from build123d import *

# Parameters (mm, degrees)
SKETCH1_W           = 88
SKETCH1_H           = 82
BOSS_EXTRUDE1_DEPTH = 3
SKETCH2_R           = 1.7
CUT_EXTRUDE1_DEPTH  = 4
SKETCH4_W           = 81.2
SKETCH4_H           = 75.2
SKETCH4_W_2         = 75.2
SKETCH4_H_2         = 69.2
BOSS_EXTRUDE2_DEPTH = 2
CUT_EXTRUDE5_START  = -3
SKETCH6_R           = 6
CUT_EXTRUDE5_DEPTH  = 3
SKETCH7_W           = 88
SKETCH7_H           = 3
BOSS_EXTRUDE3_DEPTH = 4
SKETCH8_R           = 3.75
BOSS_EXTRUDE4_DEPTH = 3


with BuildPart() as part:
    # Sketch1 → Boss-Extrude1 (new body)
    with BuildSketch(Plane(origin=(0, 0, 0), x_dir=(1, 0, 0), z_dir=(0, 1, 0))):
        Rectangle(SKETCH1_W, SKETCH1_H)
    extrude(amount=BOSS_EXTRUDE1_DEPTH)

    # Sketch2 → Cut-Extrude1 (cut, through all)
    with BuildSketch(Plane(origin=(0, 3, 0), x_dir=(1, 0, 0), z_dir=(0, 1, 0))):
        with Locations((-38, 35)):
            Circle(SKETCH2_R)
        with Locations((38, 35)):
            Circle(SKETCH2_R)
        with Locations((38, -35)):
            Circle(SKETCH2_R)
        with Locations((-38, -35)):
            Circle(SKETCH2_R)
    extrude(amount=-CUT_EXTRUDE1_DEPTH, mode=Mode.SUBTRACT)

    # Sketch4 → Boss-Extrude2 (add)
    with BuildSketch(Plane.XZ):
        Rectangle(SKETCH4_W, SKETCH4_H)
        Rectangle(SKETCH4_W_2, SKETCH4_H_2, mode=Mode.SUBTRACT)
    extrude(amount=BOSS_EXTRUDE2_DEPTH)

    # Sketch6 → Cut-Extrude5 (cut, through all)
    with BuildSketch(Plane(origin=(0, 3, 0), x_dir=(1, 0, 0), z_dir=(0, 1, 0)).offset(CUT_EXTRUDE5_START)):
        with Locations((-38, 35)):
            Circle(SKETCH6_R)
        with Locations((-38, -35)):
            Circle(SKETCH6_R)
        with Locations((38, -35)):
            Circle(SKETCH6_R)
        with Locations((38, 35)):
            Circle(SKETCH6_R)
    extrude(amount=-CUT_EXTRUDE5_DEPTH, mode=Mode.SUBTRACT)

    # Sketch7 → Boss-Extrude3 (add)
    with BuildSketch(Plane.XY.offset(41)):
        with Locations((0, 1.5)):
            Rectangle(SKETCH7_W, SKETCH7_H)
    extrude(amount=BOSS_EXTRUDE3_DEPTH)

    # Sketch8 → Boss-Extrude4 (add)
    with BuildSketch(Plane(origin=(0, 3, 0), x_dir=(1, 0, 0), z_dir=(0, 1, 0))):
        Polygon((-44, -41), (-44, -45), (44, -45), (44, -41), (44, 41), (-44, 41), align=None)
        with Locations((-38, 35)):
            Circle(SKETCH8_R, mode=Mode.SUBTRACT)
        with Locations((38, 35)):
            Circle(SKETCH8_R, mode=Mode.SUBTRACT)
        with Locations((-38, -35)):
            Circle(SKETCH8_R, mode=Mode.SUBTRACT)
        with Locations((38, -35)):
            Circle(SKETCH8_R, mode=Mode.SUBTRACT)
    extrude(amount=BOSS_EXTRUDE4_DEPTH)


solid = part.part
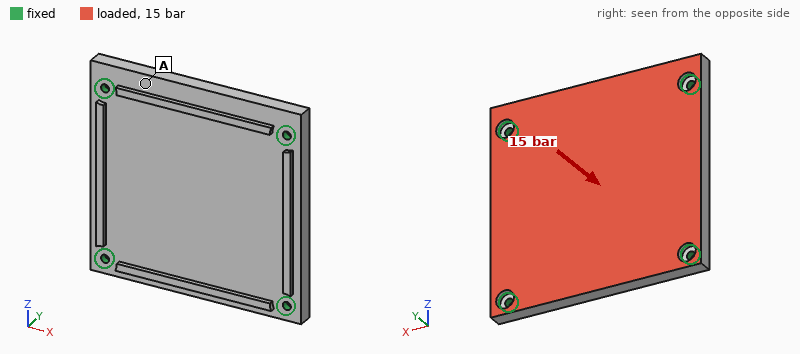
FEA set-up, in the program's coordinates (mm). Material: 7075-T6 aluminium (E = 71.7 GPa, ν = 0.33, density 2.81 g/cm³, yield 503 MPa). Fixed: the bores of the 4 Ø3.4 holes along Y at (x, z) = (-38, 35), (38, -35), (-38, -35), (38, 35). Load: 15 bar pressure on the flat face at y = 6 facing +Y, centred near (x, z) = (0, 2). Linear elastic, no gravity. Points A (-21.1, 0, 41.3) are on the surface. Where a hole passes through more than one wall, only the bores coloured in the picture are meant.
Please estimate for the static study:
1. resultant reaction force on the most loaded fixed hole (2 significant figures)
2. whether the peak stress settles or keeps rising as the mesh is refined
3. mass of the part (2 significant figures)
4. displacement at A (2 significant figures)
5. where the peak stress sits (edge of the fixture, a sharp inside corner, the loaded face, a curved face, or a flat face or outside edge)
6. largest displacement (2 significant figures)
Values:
4.4 kN
keeps rising
130 g
0.13 mm
edge of the fixture
0.35 mm
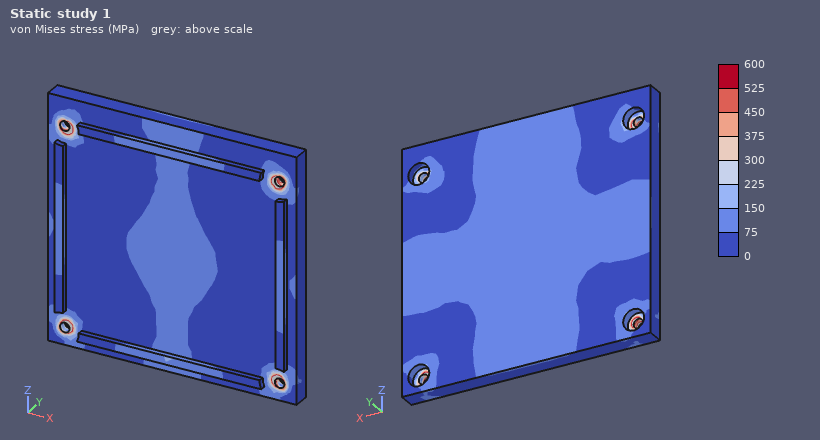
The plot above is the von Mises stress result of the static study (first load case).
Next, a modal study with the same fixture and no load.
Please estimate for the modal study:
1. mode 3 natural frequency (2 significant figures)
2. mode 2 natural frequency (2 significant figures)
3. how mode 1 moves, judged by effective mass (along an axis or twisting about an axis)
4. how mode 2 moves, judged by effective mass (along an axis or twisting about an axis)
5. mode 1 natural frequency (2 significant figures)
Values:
5300 Hz
4700 Hz
along Y
twisting about X
3000 Hz
